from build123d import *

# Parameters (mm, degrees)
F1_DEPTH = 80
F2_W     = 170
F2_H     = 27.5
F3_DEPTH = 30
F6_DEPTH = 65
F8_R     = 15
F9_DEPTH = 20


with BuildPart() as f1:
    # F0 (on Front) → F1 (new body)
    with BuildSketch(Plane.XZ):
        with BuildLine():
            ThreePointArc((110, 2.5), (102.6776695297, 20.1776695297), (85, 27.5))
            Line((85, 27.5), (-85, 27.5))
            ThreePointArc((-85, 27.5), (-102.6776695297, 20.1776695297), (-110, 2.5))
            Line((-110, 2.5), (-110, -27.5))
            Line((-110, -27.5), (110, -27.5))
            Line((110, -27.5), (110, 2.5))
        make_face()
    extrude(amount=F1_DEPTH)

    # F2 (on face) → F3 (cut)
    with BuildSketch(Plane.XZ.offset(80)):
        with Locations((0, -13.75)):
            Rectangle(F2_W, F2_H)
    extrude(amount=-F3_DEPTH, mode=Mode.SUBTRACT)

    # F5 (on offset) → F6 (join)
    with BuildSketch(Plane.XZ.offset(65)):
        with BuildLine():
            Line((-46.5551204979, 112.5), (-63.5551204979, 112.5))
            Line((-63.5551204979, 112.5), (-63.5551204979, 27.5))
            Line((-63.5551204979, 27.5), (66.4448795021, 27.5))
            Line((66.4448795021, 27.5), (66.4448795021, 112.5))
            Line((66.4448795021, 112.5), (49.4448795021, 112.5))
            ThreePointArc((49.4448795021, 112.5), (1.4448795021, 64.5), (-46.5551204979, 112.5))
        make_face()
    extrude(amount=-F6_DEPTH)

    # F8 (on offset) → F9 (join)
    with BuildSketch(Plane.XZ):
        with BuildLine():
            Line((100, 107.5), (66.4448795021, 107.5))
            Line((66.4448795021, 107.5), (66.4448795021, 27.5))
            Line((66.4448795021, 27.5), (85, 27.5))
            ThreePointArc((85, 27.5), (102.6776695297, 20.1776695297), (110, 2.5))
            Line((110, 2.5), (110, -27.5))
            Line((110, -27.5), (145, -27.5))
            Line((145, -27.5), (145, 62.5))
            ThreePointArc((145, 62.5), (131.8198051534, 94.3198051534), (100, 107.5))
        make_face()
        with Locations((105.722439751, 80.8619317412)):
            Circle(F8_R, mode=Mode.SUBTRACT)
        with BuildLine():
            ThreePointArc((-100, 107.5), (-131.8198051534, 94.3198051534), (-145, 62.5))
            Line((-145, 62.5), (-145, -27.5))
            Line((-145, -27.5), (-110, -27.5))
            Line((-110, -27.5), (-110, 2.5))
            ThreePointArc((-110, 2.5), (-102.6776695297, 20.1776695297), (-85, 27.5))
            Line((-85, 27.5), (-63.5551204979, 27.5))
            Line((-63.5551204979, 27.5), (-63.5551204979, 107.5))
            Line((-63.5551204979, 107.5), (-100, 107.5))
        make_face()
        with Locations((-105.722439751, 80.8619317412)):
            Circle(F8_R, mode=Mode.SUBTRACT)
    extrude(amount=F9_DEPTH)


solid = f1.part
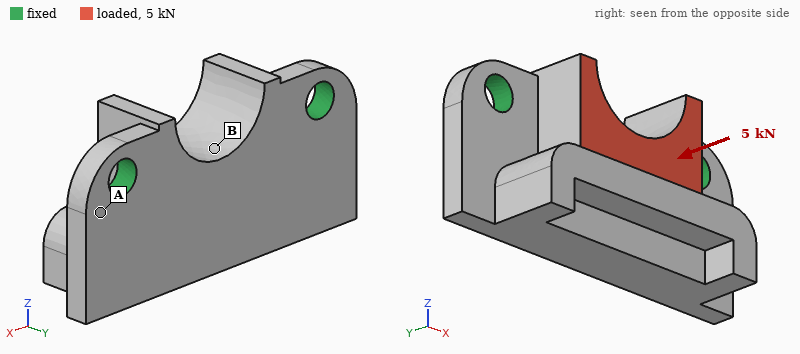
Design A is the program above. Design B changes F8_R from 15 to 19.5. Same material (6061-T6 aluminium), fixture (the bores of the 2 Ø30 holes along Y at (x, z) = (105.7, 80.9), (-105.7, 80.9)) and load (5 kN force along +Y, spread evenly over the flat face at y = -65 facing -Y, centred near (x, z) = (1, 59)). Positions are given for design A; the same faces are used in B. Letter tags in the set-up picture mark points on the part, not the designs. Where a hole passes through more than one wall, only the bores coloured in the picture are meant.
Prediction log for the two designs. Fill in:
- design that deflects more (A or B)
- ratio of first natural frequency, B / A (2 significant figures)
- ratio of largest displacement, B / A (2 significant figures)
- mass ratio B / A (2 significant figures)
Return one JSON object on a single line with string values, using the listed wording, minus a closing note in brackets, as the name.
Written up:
{"design that deflects more": "A", "ratio of first natural frequency, B / A": "1.2", "ratio of largest displacement, B / A": "0.74", "mass ratio B / A": "0.99"}
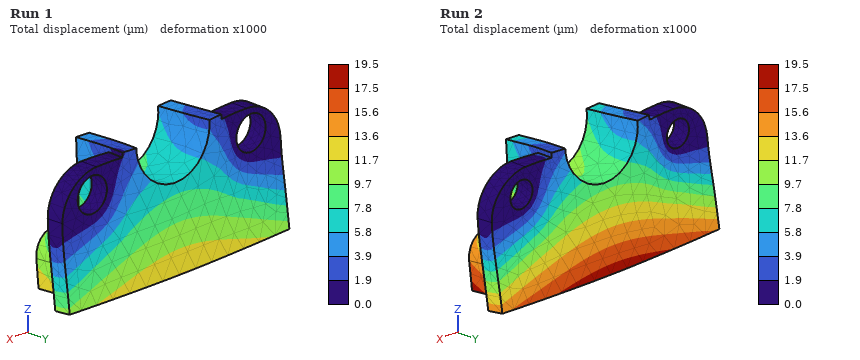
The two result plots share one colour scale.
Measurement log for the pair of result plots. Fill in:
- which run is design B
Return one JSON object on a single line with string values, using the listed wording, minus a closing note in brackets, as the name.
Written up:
{"which run is design B": "Run 1"}
